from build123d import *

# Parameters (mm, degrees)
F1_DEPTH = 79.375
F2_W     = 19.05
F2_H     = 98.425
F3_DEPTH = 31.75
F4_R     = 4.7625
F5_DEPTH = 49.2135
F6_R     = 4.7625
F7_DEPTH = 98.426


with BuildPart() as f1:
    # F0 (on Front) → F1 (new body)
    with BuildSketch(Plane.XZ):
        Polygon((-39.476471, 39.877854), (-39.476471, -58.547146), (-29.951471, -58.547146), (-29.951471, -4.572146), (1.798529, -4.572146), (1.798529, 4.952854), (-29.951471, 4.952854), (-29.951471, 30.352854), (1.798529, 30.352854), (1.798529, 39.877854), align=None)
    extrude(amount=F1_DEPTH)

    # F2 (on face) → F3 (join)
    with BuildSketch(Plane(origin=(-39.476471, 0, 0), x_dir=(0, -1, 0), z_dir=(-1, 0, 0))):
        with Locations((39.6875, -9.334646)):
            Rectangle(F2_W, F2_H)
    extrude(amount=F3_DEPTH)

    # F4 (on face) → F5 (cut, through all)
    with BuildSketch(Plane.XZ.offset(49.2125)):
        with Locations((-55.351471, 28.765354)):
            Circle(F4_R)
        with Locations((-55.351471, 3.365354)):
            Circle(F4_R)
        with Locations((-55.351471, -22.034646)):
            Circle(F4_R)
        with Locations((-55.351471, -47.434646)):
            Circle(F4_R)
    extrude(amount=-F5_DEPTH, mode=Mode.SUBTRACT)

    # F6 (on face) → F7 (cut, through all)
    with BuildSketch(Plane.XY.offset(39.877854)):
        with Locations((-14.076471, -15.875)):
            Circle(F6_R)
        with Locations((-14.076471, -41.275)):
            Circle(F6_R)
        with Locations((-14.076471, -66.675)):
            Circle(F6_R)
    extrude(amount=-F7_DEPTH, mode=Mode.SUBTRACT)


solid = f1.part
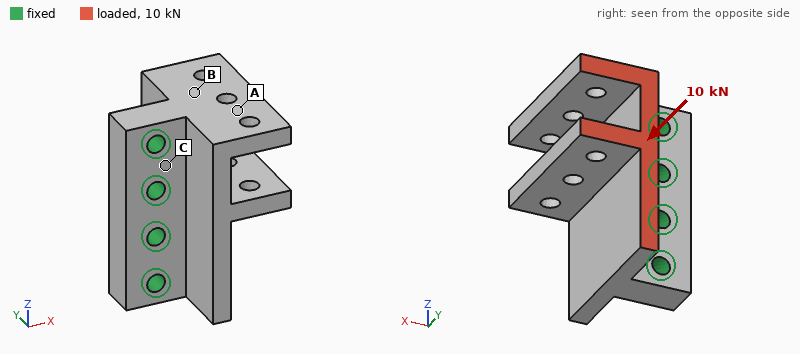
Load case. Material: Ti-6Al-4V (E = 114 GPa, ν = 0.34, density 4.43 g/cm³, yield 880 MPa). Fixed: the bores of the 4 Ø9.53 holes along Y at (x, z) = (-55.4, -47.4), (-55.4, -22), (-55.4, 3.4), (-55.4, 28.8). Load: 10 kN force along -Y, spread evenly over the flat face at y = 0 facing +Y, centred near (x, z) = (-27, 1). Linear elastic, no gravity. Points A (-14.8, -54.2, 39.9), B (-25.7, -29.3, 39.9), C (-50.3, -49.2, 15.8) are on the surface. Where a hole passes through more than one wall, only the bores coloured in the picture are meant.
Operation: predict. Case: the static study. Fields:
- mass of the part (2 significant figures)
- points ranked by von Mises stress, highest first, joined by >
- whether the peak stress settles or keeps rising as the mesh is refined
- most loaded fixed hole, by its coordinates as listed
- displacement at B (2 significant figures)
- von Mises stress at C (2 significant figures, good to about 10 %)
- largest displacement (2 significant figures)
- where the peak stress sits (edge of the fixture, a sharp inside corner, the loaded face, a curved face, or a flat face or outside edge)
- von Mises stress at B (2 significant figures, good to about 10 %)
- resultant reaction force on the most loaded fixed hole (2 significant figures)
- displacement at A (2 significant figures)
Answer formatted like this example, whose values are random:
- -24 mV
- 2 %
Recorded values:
- 760 g
- C > B > A
- keeps rising
- (-55.4, 28.8)
- 25 µm
- 26 MPa
- 66 µm
- edge of the fixture
- 13 MPa
- 3.6 kN
- 36 µm
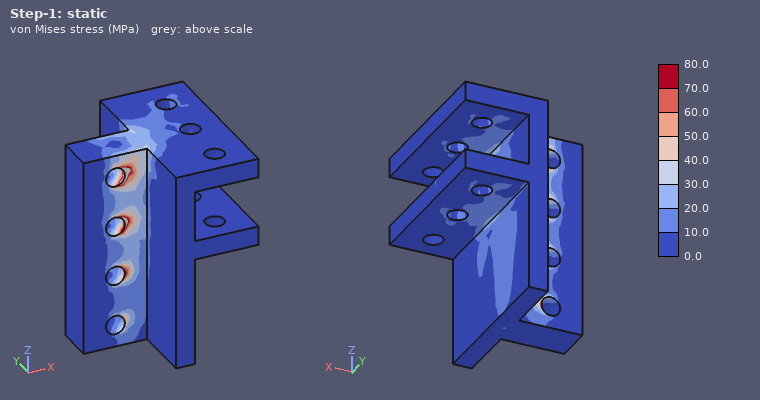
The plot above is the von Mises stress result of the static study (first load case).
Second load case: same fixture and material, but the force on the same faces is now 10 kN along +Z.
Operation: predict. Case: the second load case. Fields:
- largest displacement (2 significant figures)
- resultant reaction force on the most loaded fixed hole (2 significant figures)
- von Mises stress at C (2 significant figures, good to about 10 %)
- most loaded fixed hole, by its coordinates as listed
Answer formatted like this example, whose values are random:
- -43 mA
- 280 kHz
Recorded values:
- 0.12 mm
- 6.4 kN
- 7.2 MPa
- (-55.4, 28.8)
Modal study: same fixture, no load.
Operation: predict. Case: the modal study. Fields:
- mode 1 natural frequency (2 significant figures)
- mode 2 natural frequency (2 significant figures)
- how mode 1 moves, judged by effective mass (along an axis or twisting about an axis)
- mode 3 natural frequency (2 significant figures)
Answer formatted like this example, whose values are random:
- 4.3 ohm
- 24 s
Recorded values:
- 3200 Hz
- 4600 Hz
- along Y
- 5100 Hz
